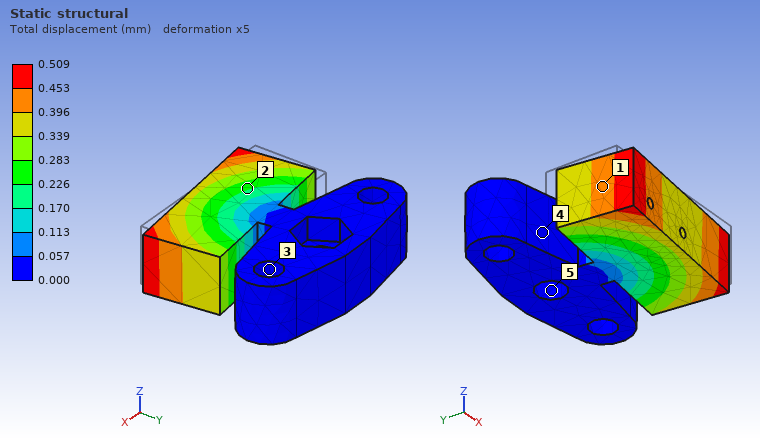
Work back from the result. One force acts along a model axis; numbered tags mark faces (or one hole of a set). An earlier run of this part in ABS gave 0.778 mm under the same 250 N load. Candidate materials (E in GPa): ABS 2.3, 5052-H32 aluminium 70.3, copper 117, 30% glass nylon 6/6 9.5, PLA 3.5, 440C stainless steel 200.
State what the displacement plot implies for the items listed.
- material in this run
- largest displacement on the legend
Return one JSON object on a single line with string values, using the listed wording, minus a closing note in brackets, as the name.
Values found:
{"material in this run": "PLA", "largest displacement on the legend": "0.509 mm"}
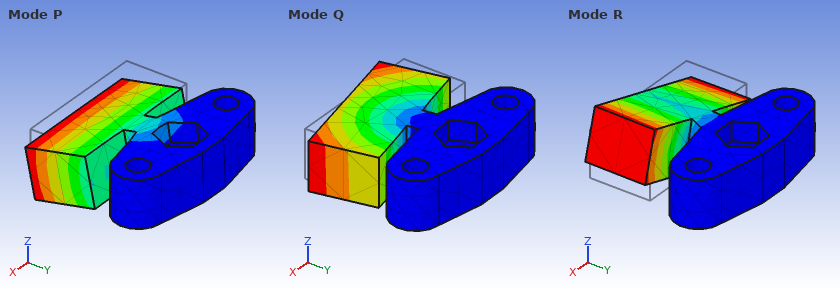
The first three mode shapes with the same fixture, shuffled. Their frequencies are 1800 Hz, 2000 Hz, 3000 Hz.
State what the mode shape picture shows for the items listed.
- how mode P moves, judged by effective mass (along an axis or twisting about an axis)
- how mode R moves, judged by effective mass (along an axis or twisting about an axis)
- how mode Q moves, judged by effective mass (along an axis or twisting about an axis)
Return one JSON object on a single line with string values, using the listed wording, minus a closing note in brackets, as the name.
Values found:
{"how mode P moves, judged by effective mass": "along Z", "how mode R moves, judged by effective mass": "twisting about Y", "how mode Q moves, judged by effective mass": "along X"}
